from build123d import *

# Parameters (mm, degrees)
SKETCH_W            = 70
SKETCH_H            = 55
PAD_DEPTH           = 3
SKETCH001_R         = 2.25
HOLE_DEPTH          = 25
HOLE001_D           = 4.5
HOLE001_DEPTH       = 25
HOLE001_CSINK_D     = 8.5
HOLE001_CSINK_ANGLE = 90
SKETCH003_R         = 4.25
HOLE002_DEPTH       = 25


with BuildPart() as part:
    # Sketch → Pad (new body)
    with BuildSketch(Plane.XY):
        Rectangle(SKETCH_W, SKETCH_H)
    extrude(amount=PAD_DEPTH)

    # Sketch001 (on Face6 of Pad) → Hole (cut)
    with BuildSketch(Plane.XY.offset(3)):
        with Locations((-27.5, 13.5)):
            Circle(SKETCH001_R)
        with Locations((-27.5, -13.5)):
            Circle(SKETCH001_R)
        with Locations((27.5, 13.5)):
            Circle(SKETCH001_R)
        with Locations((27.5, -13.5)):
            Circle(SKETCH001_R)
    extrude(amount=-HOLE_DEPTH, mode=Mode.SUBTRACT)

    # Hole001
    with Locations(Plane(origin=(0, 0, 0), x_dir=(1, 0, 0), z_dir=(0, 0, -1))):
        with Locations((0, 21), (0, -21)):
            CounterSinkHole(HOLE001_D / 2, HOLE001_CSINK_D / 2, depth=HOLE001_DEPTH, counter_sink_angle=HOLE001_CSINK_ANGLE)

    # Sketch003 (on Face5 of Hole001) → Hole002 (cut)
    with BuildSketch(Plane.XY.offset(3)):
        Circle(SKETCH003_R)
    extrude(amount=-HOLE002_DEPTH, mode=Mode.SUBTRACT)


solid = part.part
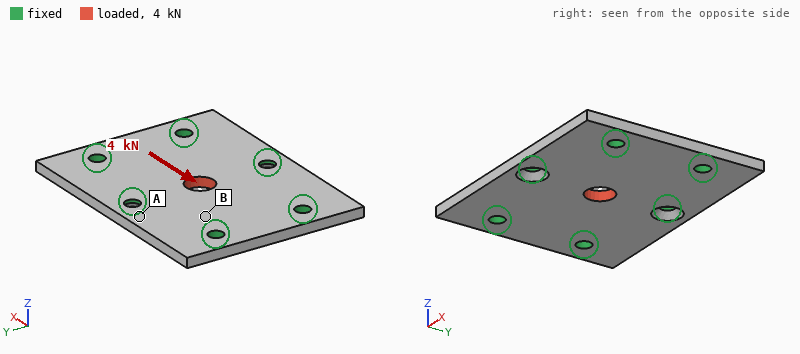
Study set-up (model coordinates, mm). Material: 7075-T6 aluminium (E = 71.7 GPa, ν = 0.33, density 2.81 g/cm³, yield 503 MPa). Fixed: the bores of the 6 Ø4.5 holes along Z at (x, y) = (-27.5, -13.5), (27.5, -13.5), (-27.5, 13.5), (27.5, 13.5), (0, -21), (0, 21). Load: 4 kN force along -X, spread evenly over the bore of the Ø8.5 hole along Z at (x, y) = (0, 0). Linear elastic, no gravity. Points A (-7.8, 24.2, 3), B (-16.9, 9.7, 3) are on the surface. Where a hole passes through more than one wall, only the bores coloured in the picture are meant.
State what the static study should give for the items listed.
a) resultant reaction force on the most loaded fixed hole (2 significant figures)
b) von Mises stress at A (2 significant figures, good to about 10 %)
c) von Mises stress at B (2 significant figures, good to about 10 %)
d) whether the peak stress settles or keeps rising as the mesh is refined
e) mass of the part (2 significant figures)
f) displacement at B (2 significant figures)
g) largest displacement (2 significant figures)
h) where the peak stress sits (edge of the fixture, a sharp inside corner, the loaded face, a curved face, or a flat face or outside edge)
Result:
820 N
8.7 MPa
21 MPa
keeps rising
31 g
3.2 µm
11 µm
edge of the fixture
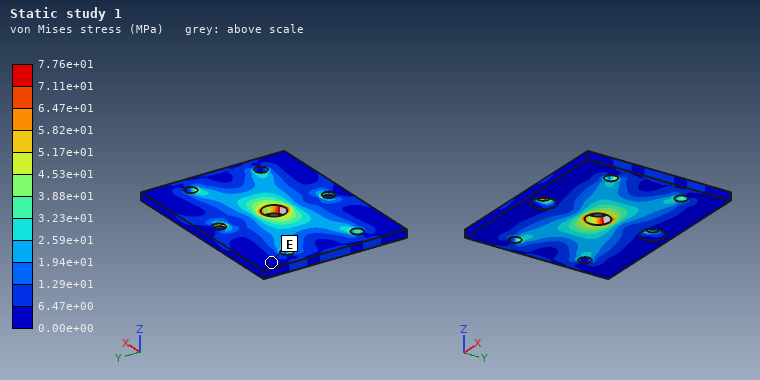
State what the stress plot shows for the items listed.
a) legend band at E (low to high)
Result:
0.00e+00 to 6.47e+00 MPa
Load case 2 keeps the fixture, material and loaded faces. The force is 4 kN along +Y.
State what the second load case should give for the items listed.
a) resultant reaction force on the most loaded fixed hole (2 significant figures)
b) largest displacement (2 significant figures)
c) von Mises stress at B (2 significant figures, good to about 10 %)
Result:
1.2 kN
12 µm
13 MPa
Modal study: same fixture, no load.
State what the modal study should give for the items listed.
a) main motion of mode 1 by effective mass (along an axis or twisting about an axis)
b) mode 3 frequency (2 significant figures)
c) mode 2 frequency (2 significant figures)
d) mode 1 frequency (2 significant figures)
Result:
along Z
13 kHz
13 kHz
9100 Hz
